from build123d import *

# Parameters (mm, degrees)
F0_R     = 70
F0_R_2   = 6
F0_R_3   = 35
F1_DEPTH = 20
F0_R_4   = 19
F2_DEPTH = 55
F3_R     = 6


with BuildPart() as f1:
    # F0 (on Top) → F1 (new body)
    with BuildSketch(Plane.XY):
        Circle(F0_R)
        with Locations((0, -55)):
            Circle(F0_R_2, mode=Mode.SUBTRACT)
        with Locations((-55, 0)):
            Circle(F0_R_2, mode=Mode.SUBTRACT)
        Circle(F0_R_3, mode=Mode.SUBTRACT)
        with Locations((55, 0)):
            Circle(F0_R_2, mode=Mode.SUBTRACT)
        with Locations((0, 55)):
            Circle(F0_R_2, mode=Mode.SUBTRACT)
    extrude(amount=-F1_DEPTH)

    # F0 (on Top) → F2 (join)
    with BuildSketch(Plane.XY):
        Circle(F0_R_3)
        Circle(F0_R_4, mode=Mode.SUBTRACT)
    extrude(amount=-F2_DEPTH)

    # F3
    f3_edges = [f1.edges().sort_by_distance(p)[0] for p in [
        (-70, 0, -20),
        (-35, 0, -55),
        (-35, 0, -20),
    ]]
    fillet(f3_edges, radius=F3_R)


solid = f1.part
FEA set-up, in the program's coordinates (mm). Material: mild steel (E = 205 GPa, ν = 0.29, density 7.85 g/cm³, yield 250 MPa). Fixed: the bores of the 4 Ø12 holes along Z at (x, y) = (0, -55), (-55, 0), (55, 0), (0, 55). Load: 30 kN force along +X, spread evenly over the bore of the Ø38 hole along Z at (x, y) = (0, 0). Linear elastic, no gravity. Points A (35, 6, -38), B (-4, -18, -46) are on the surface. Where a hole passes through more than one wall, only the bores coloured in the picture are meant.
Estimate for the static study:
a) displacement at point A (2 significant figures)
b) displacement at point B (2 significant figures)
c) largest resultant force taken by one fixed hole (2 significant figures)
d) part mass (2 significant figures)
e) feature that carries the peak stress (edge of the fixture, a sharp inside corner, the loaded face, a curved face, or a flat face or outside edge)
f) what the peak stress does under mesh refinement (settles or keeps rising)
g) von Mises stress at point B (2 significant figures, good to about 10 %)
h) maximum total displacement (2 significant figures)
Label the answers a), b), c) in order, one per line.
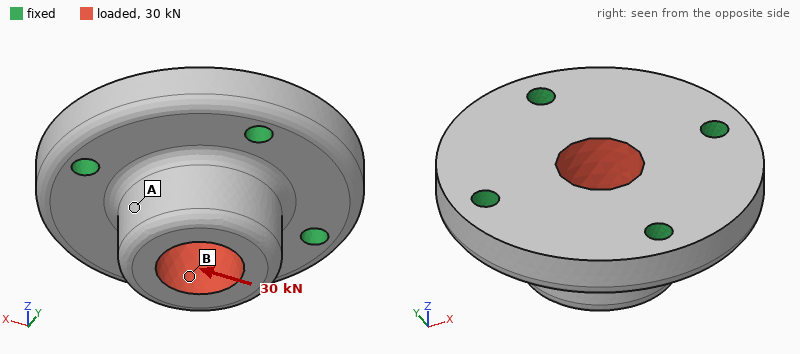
a) 5.8 µm
b) 6.3 µm
c) 11 kN
d) 2.9 kg
e) edge of the fixture
f) keeps rising
g) 14 MPa
h) 7.9 µm
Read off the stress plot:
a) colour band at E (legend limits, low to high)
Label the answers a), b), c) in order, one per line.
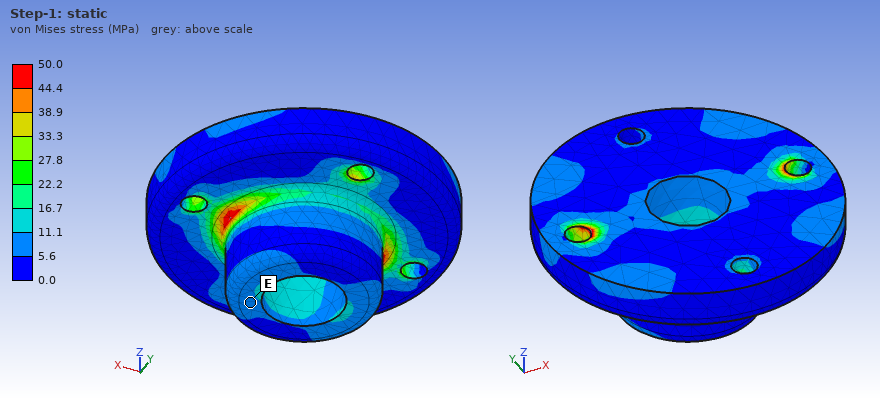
a) 5.6 to 11.1 MPa
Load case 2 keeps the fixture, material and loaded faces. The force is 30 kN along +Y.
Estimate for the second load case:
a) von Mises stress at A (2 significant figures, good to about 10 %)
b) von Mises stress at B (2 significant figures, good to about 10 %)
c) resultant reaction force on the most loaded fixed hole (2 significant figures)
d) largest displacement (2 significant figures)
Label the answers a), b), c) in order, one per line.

a) 6.3 MPa
b) 8.3 MPa
c) 11 kN
d) 7.9 µm
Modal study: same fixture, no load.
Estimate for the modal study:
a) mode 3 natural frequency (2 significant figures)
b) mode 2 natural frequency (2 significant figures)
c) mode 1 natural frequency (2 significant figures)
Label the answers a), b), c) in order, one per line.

a) 9600 Hz
b) 9500 Hz
c) 9500 Hz
